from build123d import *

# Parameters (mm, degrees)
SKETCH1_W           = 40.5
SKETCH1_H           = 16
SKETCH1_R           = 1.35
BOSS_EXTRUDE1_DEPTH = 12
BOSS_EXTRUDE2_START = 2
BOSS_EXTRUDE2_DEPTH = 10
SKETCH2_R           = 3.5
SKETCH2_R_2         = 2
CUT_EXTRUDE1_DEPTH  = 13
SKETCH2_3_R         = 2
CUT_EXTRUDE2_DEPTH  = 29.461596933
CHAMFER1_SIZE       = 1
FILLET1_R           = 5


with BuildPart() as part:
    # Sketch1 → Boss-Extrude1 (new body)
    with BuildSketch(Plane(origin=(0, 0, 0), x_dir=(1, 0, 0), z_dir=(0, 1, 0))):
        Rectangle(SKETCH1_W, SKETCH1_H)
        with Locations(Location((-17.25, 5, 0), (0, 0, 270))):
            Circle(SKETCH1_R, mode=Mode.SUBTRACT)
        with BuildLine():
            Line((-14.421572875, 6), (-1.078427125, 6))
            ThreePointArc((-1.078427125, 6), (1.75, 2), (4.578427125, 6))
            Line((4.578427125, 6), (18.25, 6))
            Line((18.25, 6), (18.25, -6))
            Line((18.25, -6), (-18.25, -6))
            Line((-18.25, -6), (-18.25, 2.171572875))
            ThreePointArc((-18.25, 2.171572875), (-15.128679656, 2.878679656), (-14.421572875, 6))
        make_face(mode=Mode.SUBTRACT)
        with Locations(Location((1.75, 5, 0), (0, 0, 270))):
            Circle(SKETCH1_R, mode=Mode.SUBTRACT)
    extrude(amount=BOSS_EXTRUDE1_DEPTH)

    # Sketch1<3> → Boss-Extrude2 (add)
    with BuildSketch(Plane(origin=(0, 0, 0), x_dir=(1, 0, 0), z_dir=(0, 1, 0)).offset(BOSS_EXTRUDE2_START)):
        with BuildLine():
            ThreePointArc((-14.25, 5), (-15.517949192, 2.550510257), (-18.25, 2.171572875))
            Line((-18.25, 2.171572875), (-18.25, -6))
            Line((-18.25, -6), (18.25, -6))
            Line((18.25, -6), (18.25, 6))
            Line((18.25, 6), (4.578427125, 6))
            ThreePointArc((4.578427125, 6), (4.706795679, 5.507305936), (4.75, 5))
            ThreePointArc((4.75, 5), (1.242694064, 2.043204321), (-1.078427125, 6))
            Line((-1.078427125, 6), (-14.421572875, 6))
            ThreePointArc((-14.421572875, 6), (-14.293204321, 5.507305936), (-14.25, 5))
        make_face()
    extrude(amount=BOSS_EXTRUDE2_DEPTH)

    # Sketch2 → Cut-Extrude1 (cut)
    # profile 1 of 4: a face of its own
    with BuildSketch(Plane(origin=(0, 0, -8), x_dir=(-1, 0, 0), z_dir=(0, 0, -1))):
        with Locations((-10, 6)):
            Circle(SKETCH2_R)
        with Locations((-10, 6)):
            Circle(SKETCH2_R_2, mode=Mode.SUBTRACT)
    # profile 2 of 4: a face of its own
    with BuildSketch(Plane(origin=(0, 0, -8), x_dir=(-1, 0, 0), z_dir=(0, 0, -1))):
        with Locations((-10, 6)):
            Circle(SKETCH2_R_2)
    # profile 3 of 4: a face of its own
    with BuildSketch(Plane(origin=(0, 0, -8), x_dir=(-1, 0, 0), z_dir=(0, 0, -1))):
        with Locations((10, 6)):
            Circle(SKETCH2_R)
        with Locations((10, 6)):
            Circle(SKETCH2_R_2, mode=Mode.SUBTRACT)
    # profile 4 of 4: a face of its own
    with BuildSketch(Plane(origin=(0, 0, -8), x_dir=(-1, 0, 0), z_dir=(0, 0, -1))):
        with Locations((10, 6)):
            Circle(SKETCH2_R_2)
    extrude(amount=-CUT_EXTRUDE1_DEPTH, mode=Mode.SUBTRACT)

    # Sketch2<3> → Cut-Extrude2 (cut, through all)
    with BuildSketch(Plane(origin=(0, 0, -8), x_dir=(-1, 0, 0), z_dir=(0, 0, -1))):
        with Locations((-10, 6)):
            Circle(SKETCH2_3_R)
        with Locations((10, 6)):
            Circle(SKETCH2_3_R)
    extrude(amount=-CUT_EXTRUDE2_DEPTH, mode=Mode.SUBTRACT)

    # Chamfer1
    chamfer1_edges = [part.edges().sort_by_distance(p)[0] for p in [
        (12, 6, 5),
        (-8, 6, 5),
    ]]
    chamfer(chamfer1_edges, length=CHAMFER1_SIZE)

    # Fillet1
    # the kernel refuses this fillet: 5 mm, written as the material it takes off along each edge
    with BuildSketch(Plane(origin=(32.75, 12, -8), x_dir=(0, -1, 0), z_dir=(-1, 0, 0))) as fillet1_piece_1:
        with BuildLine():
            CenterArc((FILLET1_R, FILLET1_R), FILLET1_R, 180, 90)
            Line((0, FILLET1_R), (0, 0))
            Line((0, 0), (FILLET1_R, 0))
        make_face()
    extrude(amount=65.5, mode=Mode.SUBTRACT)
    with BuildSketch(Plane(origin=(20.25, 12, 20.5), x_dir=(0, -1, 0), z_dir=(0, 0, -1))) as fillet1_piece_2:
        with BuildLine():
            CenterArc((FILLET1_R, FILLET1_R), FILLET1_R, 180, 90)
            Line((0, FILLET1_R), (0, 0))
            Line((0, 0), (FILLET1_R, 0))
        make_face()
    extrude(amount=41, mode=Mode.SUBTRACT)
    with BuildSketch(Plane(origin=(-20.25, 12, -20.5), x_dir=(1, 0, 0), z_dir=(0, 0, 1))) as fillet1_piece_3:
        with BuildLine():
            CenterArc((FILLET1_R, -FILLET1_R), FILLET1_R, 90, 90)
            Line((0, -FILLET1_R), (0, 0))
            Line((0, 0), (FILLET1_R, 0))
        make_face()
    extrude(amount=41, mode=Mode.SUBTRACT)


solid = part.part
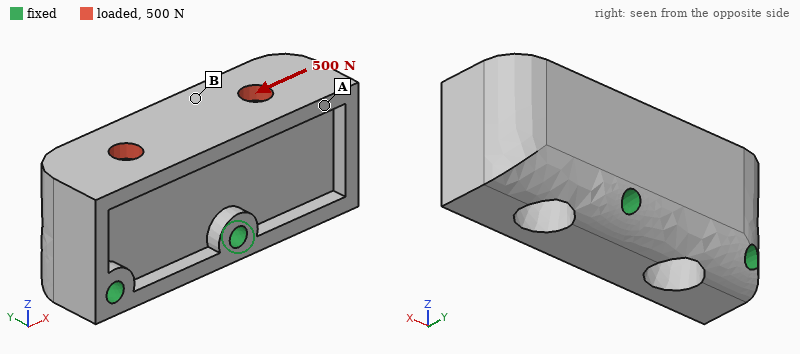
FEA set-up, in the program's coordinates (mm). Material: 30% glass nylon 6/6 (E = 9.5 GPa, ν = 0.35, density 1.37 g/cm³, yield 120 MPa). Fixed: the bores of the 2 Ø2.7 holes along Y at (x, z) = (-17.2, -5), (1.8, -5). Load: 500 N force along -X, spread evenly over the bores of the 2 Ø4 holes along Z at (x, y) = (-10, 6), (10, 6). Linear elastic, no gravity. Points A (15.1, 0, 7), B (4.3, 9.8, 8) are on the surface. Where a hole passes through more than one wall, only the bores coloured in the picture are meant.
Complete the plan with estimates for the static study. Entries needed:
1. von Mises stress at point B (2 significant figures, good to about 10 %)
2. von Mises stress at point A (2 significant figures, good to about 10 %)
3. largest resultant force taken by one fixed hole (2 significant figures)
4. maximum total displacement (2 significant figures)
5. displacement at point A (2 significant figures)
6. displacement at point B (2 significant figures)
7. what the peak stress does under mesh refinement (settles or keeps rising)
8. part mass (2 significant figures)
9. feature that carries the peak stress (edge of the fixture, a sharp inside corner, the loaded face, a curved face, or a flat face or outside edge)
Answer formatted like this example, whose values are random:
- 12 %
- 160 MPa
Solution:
- 7.1 MPa
- 2.9 MPa
- 380 N
- 44 µm
- 35 µm
- 20 µm
- keeps rising
- 7.4 g
- edge of the fixture
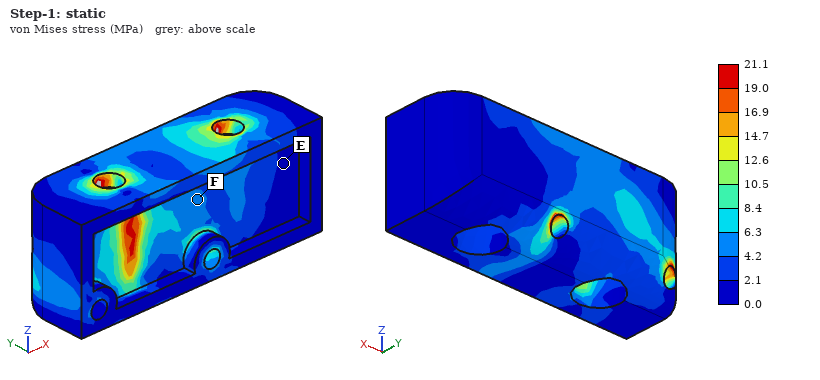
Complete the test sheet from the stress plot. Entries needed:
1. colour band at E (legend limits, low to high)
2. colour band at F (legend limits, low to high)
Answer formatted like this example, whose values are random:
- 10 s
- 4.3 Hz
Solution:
- 0.0 to 2.1 MPa
- 4.2 to 6.3 MPa
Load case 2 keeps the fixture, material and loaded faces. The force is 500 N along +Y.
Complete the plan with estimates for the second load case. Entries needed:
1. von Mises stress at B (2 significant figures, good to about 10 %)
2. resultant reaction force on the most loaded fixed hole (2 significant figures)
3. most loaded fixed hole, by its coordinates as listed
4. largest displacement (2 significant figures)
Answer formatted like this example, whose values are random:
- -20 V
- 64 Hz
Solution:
- 5.6 MPa
- 380 N
- (1.8, -5)
- 73 µm
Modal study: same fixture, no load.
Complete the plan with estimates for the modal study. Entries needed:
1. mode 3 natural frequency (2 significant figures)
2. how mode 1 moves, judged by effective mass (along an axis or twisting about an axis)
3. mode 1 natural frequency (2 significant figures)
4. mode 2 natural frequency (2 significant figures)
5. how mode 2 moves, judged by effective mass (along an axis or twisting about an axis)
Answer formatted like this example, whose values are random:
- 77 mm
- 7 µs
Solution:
- 12 kHz
- along Y
- 7000 Hz
- 8200 Hz
- along Z
